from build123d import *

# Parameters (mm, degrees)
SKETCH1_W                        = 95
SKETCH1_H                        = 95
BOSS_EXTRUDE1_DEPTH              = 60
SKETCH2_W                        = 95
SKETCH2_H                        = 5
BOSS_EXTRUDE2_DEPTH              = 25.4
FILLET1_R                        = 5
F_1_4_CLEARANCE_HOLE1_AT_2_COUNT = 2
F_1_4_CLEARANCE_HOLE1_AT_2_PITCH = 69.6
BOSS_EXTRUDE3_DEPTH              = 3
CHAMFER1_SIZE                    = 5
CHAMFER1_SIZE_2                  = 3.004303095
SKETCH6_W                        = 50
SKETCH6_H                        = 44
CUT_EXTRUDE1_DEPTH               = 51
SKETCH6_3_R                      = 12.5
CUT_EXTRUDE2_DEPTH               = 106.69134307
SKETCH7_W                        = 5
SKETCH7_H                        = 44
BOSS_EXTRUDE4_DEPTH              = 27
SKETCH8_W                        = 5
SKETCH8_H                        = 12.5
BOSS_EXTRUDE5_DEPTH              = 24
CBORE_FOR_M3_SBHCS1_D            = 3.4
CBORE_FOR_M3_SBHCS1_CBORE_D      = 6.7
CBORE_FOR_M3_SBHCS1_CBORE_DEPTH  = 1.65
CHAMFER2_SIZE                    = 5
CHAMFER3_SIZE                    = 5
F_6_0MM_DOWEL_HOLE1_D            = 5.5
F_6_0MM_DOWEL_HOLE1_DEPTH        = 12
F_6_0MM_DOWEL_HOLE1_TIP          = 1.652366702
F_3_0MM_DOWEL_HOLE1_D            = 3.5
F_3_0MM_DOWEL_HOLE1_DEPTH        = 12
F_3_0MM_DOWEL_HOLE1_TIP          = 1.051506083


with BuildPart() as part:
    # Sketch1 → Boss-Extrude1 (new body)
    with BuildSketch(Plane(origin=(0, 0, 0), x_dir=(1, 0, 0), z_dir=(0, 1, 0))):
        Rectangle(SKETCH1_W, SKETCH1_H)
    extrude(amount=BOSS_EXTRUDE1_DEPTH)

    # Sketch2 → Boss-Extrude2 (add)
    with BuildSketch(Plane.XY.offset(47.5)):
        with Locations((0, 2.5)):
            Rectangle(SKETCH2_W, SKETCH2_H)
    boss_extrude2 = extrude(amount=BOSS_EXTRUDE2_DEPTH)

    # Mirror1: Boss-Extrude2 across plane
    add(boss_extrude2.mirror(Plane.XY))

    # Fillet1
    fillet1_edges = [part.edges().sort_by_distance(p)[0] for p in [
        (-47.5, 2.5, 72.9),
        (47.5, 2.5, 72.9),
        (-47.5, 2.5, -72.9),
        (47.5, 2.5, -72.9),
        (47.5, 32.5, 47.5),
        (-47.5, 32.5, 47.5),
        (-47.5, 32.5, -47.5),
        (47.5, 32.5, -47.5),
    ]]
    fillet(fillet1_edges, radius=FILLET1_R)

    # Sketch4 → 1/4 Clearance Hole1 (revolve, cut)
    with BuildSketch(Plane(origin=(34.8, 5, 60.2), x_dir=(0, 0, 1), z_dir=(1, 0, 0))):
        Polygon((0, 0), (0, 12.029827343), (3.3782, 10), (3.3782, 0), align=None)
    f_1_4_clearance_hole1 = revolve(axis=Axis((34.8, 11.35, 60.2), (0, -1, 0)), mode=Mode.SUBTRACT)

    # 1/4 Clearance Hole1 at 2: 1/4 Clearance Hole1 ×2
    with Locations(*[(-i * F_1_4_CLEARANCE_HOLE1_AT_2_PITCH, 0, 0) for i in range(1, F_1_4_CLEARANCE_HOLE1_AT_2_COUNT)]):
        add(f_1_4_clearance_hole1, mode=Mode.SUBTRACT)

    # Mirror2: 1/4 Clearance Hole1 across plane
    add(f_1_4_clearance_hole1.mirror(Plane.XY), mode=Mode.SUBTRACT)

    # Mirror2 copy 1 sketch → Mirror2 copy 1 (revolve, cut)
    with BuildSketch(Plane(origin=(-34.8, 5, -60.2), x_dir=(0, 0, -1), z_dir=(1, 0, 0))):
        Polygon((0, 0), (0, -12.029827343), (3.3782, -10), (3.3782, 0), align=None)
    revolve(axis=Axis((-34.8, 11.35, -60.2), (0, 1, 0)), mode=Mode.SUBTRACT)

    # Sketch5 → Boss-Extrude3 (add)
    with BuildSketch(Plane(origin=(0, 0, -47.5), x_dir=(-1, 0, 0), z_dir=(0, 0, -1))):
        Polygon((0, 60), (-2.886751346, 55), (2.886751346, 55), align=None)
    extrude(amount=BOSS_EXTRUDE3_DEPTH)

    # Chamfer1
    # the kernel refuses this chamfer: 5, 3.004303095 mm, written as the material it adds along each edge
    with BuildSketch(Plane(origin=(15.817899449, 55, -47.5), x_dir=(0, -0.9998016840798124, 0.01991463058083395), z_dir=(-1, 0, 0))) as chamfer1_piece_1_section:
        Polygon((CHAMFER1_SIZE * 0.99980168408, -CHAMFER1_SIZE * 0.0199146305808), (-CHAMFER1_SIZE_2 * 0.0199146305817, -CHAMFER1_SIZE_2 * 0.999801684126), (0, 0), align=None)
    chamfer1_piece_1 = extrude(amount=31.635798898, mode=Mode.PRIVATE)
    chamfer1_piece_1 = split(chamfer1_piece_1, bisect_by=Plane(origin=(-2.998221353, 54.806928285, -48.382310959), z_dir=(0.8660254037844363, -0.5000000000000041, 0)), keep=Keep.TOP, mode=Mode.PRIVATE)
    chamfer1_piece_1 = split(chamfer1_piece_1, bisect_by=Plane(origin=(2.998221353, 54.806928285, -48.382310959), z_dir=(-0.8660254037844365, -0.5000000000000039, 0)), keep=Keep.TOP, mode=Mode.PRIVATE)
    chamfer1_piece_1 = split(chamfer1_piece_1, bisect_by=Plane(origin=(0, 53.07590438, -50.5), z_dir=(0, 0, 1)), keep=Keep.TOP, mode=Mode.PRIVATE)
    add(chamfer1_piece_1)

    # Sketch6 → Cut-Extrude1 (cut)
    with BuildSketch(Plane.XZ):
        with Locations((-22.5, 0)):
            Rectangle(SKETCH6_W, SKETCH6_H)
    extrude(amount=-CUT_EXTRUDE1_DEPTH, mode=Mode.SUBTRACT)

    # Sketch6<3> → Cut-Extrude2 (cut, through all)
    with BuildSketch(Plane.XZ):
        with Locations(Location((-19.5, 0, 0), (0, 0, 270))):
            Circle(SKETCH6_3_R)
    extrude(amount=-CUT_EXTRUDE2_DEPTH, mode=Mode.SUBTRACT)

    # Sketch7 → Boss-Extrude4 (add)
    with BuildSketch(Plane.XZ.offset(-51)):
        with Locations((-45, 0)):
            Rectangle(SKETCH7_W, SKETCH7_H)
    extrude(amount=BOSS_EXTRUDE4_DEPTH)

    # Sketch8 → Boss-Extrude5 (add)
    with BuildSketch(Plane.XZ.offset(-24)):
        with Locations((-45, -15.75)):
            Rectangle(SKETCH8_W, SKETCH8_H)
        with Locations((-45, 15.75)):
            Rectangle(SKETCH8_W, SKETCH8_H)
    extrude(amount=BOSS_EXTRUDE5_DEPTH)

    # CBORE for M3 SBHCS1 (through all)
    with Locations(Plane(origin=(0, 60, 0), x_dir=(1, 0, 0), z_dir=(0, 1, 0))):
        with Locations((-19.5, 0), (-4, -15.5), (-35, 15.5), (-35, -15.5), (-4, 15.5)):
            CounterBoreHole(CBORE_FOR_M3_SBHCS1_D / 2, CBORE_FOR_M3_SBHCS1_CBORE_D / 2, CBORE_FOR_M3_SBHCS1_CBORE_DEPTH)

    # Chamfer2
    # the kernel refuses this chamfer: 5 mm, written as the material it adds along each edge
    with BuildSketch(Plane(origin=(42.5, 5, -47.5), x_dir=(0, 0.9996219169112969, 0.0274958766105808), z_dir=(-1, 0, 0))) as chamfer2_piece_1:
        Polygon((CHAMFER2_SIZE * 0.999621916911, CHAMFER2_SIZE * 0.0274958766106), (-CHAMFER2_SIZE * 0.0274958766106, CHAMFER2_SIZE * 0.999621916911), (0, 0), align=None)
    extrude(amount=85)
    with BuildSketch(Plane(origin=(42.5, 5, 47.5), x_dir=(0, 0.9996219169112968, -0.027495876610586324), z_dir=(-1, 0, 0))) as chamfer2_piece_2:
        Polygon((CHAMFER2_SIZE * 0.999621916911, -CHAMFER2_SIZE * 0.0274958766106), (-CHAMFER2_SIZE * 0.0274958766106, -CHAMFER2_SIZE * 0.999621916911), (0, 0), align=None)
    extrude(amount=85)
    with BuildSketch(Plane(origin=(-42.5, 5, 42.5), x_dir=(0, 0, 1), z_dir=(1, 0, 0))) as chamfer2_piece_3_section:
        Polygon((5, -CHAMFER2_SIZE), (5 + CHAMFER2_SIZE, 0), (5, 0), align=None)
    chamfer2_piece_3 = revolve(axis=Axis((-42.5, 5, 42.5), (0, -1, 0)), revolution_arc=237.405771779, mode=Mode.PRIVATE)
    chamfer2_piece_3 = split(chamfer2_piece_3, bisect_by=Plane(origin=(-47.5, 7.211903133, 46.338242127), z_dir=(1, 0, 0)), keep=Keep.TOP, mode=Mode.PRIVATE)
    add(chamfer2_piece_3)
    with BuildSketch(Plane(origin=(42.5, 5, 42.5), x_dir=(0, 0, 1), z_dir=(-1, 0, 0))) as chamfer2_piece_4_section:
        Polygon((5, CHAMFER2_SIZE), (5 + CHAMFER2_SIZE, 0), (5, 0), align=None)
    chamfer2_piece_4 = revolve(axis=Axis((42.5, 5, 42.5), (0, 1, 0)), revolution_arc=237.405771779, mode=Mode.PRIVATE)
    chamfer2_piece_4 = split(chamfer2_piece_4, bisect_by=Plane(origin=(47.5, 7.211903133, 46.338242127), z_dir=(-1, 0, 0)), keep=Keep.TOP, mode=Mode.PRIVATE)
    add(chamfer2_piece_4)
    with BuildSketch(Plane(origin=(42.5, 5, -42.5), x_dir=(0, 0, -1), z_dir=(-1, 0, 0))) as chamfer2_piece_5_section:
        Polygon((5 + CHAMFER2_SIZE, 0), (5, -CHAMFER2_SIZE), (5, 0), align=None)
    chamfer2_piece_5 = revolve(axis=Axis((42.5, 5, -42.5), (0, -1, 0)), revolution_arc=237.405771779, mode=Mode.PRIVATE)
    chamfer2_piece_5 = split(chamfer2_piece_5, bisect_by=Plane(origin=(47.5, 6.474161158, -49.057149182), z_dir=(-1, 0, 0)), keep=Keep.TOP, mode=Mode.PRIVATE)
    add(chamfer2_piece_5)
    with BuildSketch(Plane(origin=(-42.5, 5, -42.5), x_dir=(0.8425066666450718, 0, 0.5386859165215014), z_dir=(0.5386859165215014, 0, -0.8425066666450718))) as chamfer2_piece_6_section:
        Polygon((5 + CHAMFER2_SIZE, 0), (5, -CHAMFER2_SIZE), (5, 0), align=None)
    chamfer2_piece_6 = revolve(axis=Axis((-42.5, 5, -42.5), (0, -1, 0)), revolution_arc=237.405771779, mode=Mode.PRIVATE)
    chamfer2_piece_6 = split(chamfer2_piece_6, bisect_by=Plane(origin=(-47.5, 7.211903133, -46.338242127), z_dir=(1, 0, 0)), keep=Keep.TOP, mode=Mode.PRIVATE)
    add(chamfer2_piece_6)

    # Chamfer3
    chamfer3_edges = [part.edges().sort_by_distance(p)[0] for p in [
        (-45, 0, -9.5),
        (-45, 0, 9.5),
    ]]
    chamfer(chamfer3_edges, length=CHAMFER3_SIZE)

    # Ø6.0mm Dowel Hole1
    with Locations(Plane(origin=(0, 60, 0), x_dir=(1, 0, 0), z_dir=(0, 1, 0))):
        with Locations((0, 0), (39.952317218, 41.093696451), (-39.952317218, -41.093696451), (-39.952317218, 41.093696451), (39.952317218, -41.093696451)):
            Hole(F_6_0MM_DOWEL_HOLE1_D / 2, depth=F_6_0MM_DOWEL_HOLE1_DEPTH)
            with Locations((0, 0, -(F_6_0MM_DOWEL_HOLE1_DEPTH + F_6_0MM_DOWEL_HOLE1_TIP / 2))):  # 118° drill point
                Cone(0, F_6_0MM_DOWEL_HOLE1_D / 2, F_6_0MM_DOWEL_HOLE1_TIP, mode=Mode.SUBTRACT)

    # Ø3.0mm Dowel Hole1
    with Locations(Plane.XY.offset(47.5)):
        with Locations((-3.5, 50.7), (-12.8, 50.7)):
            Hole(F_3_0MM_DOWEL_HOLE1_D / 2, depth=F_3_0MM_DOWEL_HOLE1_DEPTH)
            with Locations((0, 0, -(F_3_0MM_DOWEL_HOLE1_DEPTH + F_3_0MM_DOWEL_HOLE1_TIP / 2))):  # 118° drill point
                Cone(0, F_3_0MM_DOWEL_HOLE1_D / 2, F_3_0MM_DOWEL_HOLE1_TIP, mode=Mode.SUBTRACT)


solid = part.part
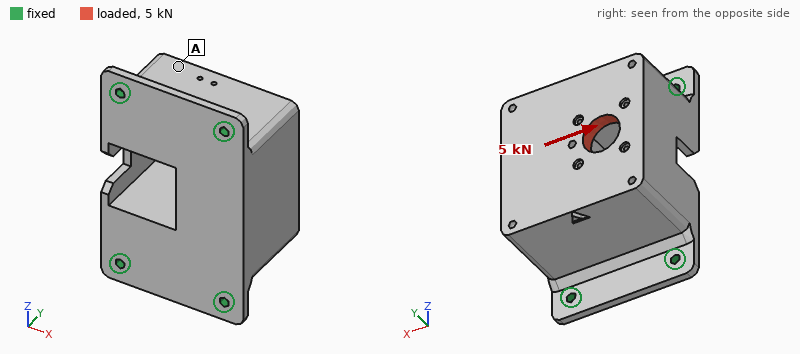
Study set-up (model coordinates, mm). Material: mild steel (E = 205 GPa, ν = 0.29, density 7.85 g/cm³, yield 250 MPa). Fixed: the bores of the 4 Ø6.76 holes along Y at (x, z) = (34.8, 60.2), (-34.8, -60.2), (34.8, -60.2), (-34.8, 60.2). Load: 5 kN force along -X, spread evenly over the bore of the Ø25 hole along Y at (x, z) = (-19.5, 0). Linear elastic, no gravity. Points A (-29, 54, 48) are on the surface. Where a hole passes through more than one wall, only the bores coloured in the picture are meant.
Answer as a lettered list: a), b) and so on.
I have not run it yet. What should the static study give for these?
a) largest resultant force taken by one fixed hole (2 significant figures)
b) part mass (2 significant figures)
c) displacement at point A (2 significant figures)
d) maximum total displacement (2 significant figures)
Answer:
a) 2.7 kN
b) 3.6 kg
c) 13 µm
d) 18 µm
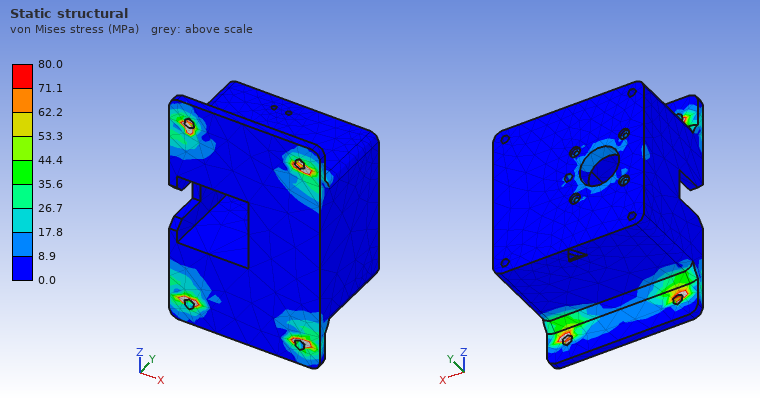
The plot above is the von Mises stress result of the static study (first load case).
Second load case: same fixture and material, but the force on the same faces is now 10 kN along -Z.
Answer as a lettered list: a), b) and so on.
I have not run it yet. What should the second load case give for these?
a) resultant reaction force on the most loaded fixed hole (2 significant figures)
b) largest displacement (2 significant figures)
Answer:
a) 3.7 kN
b) 16 µm
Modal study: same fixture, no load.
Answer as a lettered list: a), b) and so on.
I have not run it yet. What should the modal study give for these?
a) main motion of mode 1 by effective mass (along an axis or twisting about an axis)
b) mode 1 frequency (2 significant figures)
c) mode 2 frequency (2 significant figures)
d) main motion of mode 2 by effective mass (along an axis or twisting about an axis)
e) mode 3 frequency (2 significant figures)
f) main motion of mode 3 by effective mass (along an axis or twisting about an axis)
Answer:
a) along X
b) 2200 Hz
c) 2800 Hz
d) along Y
e) 3400 Hz
f) along Z
